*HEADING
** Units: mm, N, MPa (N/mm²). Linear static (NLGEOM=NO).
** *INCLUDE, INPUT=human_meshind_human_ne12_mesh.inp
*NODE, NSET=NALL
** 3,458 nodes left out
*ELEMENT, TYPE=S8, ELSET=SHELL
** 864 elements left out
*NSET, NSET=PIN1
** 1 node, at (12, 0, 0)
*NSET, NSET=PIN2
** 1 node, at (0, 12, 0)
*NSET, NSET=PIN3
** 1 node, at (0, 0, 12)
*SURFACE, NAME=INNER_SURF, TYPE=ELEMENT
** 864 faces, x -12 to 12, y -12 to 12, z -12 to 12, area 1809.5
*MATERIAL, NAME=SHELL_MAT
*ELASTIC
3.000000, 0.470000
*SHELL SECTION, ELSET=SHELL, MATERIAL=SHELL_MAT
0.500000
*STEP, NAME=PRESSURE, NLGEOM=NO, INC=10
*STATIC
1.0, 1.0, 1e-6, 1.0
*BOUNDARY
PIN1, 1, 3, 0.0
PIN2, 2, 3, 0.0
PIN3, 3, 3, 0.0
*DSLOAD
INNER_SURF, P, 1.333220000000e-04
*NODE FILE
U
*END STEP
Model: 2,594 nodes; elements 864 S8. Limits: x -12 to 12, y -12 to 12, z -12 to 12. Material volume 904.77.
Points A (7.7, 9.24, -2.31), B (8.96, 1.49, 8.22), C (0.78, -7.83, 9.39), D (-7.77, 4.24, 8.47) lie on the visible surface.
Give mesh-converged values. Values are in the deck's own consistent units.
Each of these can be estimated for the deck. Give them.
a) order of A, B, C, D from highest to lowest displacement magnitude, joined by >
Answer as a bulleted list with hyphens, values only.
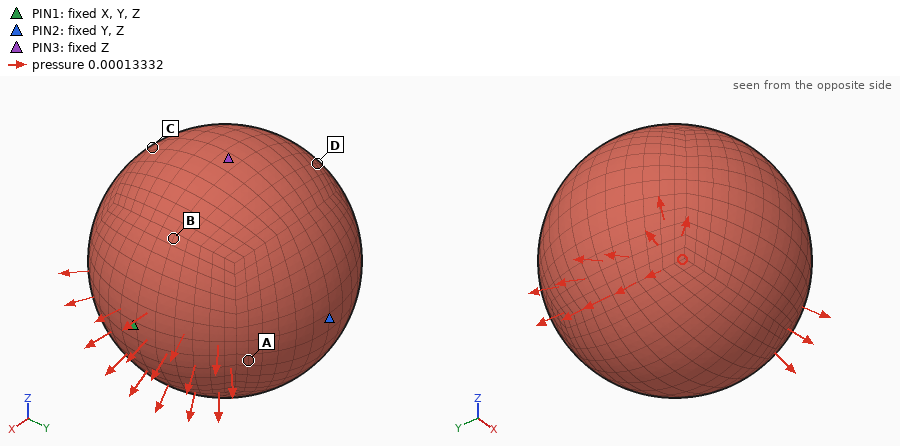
- D > C > B > A
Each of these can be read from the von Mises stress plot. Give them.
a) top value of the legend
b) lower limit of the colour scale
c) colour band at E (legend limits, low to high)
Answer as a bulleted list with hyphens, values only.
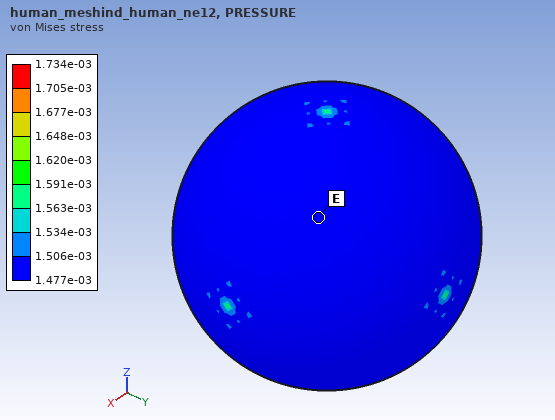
- 1.734e-03
- 1.477e-03
- 1.477e-03 to 1.506e-03
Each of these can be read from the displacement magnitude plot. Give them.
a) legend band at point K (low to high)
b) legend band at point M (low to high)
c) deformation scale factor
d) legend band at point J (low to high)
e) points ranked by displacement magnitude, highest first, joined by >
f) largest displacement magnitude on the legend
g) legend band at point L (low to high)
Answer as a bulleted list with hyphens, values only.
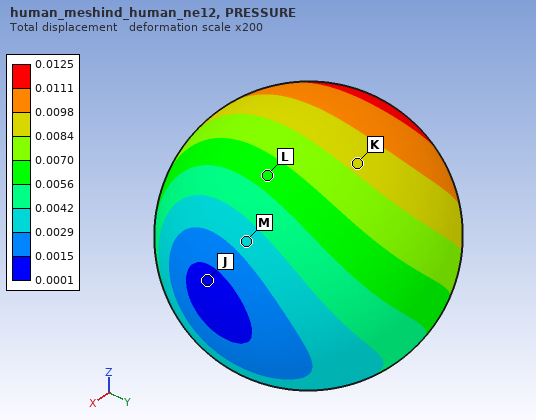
- 0.0084 to 0.0098
- 0.0029 to 0.0042
- 200
- 0.0001 to 0.0015
- K > L > M > J
- 0.0125
- 0.0056 to 0.0070
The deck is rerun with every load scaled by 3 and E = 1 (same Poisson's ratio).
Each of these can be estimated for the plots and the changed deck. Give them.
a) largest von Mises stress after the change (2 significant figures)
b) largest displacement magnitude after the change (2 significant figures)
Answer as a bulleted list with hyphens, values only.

- 0.0052
- 0.11
